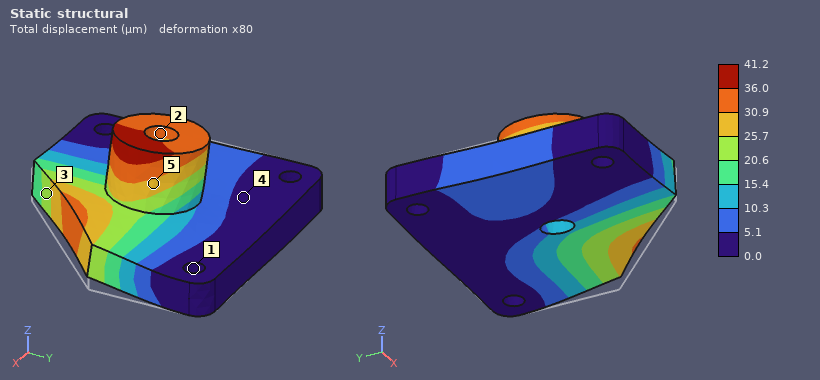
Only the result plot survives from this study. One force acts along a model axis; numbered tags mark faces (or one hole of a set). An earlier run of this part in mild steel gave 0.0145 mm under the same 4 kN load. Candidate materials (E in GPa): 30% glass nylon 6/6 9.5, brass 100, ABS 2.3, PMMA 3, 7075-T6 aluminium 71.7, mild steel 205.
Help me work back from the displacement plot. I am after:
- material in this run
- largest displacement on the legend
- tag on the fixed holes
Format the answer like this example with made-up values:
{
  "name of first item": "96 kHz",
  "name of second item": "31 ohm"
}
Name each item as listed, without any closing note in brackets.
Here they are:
{
  "material in this run": "7075-T6 aluminium",
  "largest displacement on the legend": "41.2 µm",
  "tag on the fixed holes": "1"
}
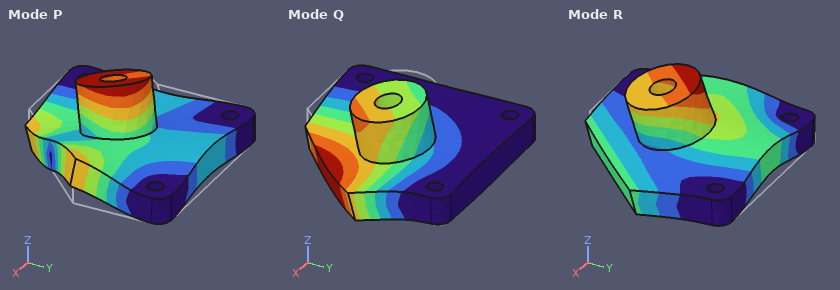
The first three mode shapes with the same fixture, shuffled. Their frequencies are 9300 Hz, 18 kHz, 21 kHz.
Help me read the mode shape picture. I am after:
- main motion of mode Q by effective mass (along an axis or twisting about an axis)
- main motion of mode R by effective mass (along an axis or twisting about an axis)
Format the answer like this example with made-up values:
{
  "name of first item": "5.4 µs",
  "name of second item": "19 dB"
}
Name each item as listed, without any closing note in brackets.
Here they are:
{
  "main motion of mode Q by effective mass": "along Z",
  "main motion of mode R by effective mass": "along Z"
}
